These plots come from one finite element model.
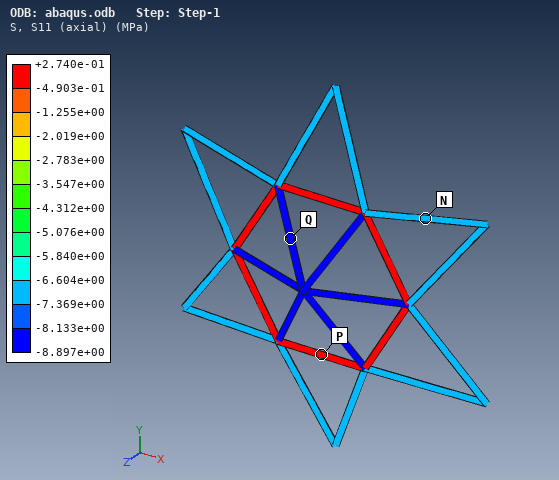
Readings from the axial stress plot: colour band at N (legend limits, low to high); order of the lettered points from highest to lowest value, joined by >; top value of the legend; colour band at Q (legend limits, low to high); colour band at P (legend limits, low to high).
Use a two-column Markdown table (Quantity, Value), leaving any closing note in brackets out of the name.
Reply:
| Quantity | Value |
|---|---|
| colour band at N | -7.369e+00 to -6.604e+00 MPa |
| order of the lettered points from highest to lowest value, joined by > | P > N > Q |
| top value of the legend | +2.740e-01 MPa |
| colour band at Q | -8.897e+00 to -8.133e+00 MPa |
| colour band at P | -4.903e-01 to +2.740e-01 MPa |
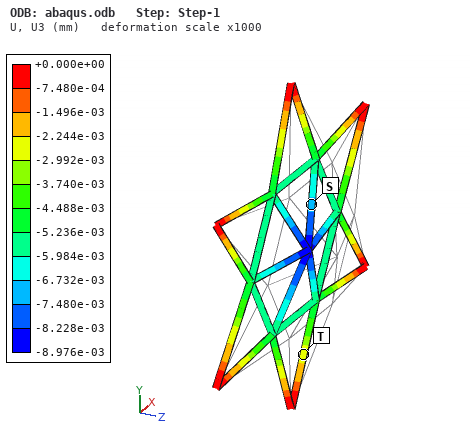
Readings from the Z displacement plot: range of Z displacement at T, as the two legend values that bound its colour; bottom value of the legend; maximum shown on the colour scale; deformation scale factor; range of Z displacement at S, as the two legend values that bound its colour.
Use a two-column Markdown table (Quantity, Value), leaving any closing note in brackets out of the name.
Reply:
| Quantity | Value |
|---|---|
| range of Z displacement at T, as the two legend values that bound its colour | -2.992e-03 to -2.244e-03 mm |
| bottom value of the legend | -8.976e-03 mm |
| maximum shown on the colour scale | +0.000e+00 mm |
| deformation scale factor | 1000 |
| range of Z displacement at S, as the two legend values that bound its colour | -7.480e-03 to -6.732e-03 mm |
